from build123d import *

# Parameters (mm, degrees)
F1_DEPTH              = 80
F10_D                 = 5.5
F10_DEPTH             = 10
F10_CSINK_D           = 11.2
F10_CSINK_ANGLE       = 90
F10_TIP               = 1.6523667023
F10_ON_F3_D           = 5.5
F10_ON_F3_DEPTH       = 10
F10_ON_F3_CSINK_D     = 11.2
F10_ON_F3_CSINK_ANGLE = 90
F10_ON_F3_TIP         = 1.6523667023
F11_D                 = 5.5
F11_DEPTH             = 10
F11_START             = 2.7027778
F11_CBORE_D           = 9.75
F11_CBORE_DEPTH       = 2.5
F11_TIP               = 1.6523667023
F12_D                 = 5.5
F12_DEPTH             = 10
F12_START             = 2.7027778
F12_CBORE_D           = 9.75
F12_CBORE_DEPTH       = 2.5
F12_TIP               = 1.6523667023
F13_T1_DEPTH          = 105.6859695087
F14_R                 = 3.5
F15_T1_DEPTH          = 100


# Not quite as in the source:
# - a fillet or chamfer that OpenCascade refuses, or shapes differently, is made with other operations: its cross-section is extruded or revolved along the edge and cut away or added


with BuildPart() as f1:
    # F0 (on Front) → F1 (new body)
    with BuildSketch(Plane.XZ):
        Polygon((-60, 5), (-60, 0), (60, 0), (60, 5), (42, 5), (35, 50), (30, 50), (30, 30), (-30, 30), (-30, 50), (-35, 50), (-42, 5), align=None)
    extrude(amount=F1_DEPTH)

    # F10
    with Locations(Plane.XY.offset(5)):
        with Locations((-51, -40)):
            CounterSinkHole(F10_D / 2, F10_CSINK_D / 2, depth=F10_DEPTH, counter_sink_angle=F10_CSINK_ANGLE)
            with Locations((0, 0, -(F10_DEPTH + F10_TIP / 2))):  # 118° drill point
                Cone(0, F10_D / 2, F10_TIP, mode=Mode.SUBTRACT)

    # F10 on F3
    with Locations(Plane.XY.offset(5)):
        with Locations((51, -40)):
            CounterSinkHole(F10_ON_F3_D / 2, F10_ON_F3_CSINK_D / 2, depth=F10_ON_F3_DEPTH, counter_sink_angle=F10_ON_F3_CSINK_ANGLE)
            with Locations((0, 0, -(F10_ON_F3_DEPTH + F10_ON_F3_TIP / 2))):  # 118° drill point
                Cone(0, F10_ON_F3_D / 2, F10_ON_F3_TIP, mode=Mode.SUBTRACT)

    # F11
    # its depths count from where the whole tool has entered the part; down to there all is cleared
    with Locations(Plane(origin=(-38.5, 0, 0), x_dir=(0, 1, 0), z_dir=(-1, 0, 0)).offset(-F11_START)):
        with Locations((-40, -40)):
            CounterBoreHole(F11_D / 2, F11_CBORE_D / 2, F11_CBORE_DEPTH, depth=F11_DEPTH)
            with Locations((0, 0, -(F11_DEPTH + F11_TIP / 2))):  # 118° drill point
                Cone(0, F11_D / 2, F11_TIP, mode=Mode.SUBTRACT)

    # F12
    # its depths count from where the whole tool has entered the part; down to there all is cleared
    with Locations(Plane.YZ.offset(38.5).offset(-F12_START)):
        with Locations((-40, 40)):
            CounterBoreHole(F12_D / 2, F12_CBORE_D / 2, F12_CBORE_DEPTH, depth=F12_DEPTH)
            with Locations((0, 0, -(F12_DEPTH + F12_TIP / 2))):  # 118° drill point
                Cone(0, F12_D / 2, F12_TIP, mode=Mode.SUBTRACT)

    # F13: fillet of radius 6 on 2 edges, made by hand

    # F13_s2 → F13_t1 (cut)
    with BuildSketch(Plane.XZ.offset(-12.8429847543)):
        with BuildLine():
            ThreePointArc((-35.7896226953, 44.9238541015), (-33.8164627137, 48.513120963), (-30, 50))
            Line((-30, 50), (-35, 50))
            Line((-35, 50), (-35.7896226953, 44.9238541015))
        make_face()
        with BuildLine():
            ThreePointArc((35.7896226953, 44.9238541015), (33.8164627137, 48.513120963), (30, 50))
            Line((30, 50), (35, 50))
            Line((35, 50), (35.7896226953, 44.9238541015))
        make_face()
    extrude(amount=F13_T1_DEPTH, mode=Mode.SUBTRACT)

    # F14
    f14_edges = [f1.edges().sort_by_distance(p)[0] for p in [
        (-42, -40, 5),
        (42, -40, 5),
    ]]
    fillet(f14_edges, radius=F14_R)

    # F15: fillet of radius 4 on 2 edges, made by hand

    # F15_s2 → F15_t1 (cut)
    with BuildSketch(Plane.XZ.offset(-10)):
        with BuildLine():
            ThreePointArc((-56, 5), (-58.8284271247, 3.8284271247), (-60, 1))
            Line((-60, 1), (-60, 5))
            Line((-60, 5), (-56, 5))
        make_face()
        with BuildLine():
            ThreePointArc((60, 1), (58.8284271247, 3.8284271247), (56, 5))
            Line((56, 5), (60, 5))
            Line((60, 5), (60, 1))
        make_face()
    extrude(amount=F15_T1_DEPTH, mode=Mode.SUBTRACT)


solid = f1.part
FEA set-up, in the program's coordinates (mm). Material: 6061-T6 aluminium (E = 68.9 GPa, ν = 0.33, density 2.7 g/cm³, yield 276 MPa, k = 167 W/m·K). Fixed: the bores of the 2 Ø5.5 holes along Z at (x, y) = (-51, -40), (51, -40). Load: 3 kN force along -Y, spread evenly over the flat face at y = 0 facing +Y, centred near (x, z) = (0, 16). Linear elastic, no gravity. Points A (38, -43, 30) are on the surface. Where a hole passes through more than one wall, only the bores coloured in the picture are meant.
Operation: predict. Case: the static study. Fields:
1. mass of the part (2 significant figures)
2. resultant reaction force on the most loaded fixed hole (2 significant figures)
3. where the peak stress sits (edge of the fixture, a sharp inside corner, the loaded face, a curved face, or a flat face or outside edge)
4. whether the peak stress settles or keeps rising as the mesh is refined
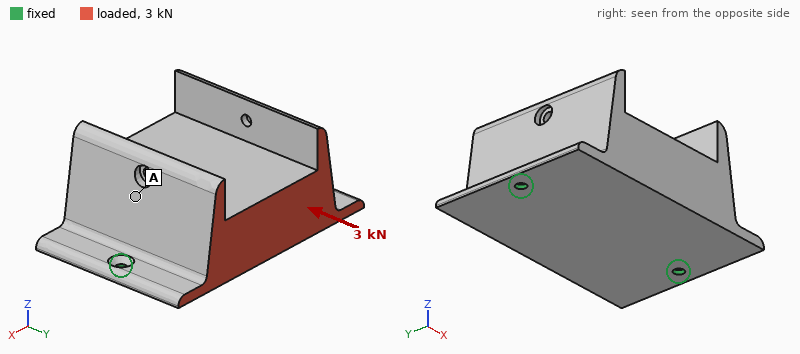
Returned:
610 g
1.5 kN
edge of the fixture
keeps rising
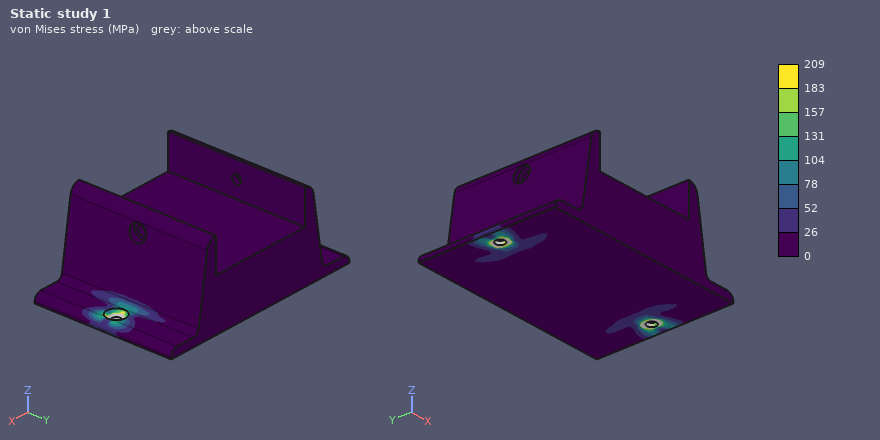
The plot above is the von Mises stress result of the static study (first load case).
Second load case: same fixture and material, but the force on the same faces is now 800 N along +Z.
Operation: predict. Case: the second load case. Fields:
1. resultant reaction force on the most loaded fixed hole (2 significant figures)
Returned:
560 N
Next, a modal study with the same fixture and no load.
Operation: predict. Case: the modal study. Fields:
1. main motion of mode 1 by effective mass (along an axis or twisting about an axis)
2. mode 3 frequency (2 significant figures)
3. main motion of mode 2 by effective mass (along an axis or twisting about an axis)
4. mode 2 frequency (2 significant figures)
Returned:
along Y
3800 Hz
along Z
2500 Hz
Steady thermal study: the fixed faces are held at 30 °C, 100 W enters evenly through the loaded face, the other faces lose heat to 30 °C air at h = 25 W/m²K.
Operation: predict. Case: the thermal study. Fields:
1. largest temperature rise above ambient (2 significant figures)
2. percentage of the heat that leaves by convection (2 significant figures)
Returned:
33 K
20 %
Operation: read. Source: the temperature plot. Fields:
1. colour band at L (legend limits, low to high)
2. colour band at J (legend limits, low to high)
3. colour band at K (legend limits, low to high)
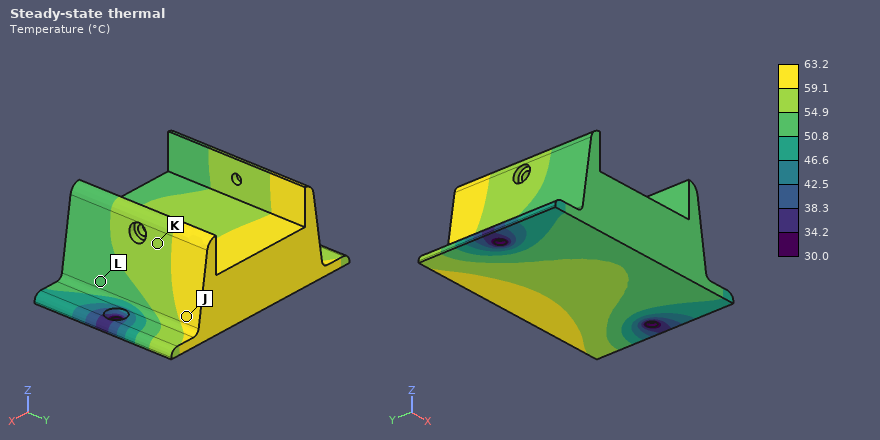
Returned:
50.8 to 54.9 °C
59.1 to 63.2 °C
54.9 to 59.1 °C
